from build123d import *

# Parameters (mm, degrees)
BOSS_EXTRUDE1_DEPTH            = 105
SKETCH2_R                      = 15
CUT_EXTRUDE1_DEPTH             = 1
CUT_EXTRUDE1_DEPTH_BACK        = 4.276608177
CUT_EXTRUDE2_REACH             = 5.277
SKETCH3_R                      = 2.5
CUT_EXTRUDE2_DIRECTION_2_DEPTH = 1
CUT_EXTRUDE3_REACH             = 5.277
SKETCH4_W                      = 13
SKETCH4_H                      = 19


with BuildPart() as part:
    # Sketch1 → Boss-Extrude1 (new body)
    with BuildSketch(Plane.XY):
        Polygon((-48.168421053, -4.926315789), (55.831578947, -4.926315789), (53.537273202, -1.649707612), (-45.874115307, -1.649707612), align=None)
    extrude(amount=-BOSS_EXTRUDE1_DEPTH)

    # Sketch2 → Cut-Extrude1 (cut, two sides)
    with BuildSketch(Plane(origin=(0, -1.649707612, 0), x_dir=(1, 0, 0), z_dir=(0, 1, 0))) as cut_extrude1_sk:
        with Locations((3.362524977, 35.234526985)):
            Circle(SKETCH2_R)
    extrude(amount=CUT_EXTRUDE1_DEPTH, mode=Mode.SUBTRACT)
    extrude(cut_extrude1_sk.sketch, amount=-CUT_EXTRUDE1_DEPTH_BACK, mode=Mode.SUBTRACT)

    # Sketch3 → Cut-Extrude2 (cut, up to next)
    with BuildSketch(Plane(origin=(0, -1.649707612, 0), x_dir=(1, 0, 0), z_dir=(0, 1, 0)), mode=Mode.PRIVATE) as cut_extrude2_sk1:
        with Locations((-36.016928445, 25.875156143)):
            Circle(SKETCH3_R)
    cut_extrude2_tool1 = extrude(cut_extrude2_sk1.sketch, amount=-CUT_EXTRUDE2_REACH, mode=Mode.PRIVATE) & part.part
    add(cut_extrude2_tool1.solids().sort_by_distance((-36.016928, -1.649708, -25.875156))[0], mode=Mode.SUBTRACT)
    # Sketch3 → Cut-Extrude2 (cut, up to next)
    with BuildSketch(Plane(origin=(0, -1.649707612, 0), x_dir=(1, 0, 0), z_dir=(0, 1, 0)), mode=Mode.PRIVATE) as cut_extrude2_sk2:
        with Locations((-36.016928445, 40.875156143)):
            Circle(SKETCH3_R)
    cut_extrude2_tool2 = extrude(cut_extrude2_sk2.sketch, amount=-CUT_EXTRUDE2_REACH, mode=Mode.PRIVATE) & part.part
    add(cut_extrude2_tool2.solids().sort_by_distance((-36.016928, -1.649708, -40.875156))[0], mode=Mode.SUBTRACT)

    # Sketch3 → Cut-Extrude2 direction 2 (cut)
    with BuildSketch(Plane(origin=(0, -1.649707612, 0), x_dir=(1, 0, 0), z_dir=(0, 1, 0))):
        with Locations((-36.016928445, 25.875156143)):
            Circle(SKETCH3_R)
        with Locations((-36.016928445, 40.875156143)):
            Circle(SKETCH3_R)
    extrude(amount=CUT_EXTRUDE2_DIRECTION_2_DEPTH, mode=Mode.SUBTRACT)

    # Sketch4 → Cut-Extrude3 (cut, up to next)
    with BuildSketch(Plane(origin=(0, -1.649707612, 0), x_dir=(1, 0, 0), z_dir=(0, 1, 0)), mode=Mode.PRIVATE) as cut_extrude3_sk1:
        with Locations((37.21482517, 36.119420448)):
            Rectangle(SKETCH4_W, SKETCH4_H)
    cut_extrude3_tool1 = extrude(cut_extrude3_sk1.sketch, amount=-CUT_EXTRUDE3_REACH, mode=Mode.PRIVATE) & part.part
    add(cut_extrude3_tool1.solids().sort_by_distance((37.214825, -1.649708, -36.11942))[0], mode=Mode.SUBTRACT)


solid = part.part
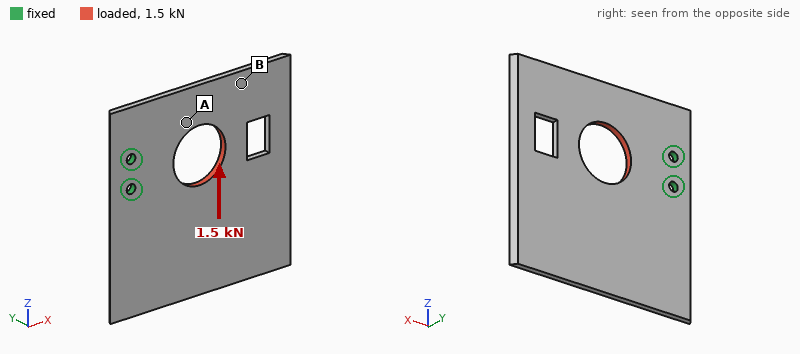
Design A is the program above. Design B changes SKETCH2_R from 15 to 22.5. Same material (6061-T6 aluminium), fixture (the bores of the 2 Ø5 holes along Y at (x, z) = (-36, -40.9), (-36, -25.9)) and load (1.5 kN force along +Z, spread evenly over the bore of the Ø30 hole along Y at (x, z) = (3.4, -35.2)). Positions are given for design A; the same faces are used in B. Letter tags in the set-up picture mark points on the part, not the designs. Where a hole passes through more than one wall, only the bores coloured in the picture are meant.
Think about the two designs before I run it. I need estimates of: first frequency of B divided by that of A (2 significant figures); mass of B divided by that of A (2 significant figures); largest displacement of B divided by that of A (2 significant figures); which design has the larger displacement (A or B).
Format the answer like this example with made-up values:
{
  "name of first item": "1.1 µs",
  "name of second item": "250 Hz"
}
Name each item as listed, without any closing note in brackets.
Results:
{
  "first frequency of B divided by that of A": "0.89",
  "mass of B divided by that of A": "0.91",
  "largest displacement of B divided by that of A": "1.4",
  "which design has the larger displacement": "B"
}
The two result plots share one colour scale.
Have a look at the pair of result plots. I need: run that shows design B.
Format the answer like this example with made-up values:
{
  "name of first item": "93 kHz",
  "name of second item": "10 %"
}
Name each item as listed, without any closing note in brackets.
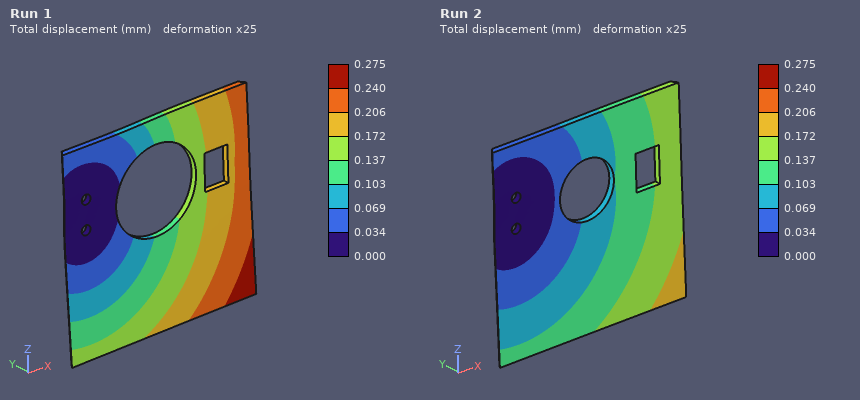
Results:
{
  "run that shows design B": "Run 1"
}
